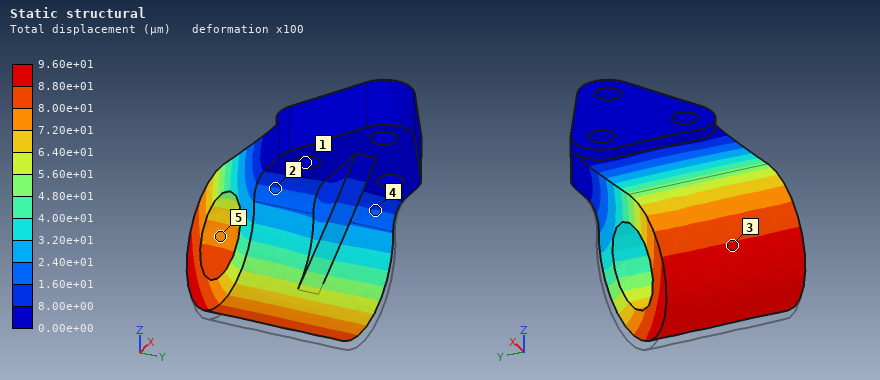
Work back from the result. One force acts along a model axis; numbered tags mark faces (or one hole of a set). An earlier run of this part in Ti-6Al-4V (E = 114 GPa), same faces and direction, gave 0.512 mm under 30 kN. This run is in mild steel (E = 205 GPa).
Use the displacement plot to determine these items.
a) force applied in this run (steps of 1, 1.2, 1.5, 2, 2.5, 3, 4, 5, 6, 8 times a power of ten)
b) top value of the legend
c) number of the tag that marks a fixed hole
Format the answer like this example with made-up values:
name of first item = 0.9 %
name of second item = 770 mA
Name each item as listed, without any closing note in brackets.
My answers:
force applied in this run = 10 kN
top value of the legend = 9.60e+01 µm
number of the tag that marks a fixed hole = 1
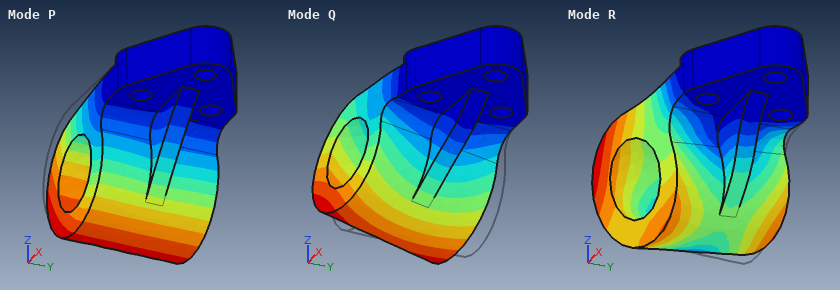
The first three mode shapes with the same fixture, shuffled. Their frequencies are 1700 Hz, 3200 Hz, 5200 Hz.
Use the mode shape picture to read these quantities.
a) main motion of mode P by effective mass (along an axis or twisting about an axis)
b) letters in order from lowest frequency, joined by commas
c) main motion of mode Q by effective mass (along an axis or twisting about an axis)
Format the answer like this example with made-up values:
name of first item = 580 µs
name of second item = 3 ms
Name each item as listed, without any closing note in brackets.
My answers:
main motion of mode P by effective mass = along Z
letters in order from lowest frequency, joined by commas = P, Q, R
main motion of mode Q by effective mass = along Y
